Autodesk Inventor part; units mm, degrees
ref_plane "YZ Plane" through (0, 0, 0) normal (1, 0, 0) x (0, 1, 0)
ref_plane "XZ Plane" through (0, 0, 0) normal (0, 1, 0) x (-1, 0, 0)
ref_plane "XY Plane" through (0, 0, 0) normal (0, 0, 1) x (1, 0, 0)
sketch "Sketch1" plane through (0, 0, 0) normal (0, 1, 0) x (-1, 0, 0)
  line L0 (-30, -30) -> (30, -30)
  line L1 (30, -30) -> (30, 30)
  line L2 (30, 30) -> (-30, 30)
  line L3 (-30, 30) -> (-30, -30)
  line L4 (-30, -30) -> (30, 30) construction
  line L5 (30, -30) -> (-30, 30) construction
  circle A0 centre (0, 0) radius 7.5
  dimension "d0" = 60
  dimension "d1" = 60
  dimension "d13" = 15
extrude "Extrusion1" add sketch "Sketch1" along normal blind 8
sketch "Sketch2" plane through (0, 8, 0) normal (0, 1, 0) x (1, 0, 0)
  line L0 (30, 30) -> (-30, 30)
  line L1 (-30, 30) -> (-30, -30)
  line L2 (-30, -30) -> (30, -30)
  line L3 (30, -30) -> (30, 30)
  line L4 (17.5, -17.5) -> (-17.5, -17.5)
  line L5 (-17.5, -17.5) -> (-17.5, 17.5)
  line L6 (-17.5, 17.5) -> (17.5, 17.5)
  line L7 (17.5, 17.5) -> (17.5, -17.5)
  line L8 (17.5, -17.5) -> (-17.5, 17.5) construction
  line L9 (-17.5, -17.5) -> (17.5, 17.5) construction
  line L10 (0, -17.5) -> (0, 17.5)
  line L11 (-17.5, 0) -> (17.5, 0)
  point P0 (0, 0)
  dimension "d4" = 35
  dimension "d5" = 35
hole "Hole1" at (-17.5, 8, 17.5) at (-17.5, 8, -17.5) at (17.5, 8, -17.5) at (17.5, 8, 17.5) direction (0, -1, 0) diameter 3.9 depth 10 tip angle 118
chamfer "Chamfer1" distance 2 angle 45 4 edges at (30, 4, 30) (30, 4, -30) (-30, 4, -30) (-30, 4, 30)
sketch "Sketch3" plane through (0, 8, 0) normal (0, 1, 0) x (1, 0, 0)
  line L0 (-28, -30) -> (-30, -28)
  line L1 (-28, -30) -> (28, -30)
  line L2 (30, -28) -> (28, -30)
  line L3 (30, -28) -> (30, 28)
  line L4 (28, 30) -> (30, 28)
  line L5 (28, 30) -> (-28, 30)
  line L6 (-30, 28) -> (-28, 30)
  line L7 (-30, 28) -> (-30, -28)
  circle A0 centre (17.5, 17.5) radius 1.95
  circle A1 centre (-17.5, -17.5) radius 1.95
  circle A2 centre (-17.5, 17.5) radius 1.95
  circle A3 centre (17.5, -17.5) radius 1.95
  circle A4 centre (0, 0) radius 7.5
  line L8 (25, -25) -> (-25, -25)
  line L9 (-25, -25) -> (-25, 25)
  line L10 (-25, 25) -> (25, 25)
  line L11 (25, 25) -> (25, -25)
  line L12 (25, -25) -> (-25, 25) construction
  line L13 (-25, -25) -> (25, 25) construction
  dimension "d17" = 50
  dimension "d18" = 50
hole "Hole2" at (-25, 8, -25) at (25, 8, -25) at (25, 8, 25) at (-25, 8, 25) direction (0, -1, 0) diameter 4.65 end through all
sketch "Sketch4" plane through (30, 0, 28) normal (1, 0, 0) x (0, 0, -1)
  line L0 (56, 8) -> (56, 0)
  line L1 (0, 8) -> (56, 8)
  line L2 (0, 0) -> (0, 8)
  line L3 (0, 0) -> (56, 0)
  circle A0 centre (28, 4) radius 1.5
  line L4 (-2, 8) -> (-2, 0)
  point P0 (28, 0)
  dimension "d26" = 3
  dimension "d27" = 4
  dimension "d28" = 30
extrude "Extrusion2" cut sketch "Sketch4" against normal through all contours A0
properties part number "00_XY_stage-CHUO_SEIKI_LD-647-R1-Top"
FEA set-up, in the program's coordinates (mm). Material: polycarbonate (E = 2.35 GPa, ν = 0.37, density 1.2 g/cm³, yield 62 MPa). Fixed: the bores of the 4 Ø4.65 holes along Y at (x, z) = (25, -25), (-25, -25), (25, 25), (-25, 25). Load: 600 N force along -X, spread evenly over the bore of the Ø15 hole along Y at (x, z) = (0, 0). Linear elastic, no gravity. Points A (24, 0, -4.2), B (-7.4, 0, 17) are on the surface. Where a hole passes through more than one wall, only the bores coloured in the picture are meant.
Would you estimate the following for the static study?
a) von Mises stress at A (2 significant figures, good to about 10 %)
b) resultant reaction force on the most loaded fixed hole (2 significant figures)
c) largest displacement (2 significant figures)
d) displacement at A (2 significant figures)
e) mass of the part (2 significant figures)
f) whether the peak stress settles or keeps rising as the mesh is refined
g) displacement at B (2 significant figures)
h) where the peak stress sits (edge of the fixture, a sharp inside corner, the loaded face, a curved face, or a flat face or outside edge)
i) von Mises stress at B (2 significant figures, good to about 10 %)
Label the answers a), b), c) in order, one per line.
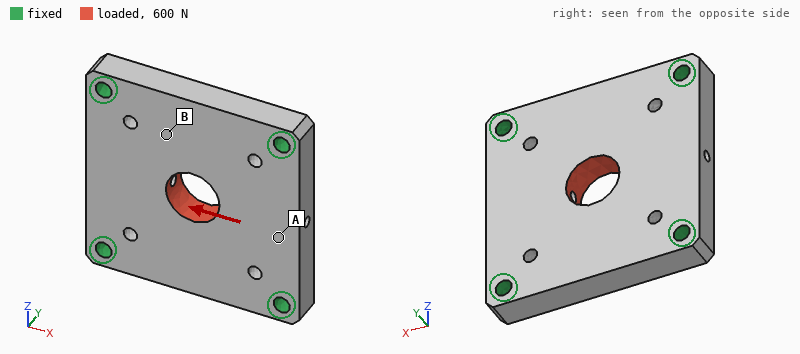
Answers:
a) 0.49 MPa
b) 170 N
c) 26 µm
d) 19 µm
e) 31 g
f) keeps rising
g) 12 µm
h) edge of the fixture
i) 1.2 MPa
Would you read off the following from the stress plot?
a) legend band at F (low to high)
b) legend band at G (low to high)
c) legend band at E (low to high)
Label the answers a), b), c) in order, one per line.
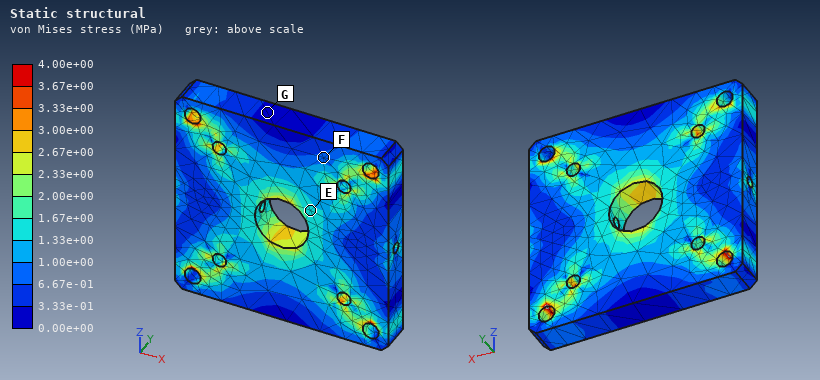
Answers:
a) 6.67e-01 to 1.00e+00 MPa
b) 0.00e+00 to 3.33e-01 MPa
c) 1.33e+00 to 1.67e+00 MPa
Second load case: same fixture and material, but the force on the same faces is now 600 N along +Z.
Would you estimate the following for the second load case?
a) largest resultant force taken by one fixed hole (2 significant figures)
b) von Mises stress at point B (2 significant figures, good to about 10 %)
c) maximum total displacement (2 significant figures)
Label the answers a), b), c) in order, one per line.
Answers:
a) 170 N
b) 1.2 MPa
c) 27 µm
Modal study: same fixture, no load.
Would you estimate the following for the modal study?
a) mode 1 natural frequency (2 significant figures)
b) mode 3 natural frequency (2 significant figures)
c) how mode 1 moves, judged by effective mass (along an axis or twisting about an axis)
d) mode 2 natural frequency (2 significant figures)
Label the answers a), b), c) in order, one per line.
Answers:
a) 2800 Hz
b) 4400 Hz
c) along Y
d) 4300 Hz
